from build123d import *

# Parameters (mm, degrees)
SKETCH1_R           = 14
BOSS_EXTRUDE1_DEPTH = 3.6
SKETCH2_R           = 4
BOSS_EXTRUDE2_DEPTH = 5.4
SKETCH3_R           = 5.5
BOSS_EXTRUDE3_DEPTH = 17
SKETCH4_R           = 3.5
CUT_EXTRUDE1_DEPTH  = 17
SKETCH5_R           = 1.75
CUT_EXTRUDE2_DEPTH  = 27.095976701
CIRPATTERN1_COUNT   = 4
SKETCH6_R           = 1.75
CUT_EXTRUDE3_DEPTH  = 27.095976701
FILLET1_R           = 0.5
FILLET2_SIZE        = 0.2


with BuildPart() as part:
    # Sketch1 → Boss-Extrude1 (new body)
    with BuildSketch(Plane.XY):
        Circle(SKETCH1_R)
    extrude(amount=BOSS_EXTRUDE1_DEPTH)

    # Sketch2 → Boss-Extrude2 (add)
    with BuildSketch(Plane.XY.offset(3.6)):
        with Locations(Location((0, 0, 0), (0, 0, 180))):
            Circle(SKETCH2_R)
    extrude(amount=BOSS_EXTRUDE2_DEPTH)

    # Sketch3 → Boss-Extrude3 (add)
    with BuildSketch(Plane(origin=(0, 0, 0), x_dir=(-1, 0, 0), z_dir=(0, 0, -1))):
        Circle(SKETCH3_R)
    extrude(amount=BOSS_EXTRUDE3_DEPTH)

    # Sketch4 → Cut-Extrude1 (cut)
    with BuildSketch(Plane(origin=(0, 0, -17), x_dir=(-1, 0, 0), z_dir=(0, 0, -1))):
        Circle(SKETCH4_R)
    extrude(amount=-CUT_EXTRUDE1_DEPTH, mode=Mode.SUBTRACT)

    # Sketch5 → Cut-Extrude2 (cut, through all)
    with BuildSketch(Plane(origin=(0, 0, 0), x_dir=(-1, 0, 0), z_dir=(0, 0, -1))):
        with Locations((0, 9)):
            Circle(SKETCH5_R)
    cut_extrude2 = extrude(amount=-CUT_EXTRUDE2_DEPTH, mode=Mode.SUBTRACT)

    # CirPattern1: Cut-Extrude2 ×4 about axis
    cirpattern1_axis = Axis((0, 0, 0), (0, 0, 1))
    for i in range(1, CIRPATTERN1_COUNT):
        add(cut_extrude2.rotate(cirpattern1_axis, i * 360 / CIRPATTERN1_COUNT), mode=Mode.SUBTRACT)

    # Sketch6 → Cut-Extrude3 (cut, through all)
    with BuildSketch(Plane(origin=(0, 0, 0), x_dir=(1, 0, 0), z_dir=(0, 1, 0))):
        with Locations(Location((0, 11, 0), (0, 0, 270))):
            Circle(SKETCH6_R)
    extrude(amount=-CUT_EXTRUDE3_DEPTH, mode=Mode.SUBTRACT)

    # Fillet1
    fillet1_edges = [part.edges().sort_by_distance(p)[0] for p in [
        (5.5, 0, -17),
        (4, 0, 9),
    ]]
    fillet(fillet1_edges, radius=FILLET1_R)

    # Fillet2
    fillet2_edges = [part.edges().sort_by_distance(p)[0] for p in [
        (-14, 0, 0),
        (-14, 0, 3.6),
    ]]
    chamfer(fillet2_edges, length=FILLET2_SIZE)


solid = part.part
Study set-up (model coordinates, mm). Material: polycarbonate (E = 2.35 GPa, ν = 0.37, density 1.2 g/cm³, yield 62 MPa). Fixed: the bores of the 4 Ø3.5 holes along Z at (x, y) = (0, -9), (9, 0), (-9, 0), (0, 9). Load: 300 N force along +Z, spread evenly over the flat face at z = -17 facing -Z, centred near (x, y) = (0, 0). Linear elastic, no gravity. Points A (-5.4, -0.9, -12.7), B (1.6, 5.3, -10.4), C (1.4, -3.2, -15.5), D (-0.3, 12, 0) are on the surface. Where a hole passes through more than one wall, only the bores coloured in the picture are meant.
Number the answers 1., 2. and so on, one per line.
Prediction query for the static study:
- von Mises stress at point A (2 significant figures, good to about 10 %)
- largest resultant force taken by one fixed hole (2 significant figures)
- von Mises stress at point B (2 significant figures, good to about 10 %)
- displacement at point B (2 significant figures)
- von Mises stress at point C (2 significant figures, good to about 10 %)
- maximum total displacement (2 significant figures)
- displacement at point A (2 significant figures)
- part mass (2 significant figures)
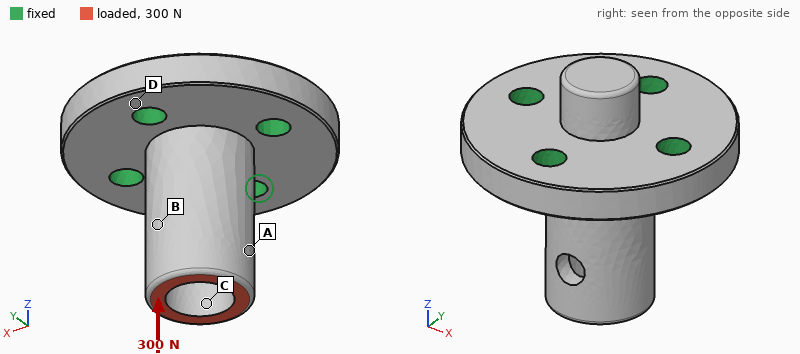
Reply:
1. 4.5 MPa
2. 77 N
3. 5.3 MPa
4. 37 µm
5. 7.5 MPa
6. 67 µm
7. 45 µm
8. 3.9 g
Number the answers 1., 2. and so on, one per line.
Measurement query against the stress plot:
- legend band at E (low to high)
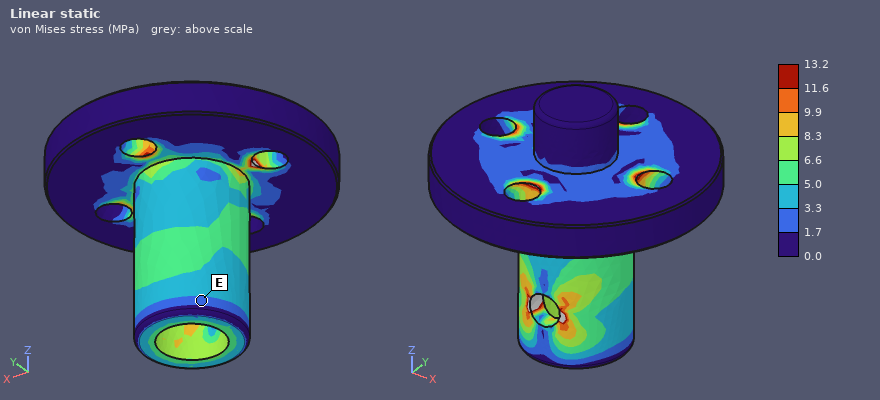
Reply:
1. 1.7 to 3.3 MPa
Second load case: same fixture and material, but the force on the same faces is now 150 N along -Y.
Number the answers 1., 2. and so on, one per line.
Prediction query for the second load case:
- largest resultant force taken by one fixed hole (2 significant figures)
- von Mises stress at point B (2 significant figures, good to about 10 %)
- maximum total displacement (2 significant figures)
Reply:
1. 190 N
2. 9.5 MPa
3. 0.42 mm
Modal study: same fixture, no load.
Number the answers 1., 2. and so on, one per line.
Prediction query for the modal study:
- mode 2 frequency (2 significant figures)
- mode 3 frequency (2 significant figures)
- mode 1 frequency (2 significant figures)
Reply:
1. 5200 Hz
2. 11 kHz
3. 5200 Hz
